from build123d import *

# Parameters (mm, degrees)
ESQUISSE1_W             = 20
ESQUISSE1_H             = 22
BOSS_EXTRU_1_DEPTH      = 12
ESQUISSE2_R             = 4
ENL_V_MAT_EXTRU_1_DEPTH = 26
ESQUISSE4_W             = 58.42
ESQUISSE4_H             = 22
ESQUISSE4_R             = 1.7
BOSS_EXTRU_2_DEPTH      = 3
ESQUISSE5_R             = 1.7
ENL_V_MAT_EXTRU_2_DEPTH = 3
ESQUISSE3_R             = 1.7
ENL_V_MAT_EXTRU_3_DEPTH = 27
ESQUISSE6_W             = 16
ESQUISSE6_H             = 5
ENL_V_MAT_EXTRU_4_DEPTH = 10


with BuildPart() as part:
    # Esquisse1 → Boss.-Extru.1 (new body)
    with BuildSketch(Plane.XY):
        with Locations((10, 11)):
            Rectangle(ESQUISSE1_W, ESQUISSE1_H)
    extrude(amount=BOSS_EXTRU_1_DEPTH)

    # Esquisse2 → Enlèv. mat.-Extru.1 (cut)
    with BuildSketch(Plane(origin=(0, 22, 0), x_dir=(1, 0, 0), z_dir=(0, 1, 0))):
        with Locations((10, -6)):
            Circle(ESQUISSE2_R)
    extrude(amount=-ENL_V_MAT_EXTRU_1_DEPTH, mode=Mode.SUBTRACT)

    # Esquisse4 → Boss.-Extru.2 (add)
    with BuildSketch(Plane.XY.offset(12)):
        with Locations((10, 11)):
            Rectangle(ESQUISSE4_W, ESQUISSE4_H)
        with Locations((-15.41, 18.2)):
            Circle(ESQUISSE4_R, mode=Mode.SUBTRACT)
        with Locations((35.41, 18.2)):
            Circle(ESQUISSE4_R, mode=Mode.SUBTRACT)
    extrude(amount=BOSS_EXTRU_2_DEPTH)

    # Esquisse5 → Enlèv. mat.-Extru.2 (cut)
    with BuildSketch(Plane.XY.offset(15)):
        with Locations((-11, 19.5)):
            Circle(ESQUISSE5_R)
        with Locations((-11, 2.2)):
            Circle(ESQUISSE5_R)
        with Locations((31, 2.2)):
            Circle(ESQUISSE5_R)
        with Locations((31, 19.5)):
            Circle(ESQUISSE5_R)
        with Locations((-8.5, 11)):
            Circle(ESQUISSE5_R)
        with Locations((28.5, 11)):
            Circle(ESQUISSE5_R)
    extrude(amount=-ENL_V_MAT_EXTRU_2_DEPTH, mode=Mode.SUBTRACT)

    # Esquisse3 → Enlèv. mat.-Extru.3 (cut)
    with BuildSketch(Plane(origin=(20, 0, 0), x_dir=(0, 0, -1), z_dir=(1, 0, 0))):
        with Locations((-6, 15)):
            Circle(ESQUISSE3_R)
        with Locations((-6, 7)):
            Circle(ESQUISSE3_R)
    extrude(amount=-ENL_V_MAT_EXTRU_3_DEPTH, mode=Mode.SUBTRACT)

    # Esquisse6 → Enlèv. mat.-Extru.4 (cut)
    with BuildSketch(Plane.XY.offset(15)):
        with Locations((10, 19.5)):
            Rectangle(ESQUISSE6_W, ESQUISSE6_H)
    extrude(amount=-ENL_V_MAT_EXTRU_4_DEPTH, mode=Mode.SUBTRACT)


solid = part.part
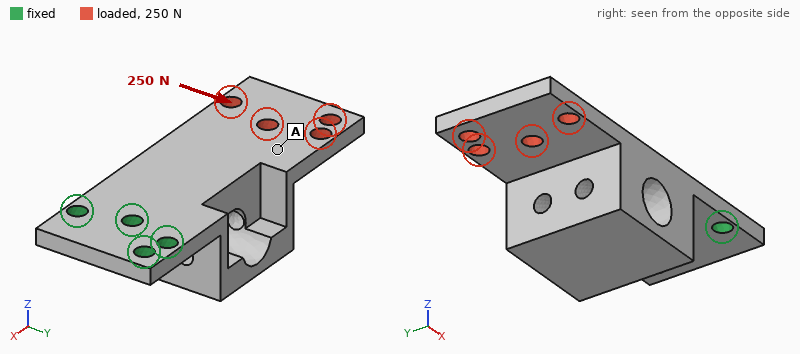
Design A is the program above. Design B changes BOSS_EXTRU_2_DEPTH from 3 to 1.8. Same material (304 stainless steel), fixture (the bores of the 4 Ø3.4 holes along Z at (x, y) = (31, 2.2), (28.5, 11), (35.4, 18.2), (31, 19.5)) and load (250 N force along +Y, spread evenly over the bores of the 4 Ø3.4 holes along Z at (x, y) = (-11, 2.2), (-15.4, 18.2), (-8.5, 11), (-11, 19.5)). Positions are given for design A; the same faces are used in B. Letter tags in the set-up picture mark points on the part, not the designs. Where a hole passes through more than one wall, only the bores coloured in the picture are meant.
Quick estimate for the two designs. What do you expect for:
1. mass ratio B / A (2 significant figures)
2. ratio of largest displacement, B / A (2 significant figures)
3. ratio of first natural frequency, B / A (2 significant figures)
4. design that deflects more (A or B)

0.80
1.5
0.57
B
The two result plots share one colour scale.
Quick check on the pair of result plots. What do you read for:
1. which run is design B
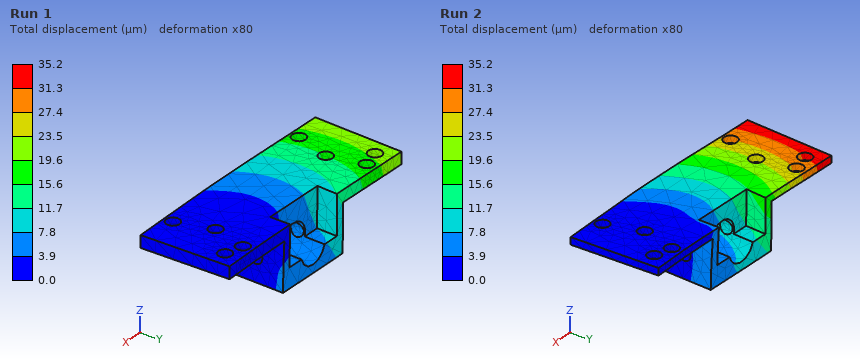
Run 2
